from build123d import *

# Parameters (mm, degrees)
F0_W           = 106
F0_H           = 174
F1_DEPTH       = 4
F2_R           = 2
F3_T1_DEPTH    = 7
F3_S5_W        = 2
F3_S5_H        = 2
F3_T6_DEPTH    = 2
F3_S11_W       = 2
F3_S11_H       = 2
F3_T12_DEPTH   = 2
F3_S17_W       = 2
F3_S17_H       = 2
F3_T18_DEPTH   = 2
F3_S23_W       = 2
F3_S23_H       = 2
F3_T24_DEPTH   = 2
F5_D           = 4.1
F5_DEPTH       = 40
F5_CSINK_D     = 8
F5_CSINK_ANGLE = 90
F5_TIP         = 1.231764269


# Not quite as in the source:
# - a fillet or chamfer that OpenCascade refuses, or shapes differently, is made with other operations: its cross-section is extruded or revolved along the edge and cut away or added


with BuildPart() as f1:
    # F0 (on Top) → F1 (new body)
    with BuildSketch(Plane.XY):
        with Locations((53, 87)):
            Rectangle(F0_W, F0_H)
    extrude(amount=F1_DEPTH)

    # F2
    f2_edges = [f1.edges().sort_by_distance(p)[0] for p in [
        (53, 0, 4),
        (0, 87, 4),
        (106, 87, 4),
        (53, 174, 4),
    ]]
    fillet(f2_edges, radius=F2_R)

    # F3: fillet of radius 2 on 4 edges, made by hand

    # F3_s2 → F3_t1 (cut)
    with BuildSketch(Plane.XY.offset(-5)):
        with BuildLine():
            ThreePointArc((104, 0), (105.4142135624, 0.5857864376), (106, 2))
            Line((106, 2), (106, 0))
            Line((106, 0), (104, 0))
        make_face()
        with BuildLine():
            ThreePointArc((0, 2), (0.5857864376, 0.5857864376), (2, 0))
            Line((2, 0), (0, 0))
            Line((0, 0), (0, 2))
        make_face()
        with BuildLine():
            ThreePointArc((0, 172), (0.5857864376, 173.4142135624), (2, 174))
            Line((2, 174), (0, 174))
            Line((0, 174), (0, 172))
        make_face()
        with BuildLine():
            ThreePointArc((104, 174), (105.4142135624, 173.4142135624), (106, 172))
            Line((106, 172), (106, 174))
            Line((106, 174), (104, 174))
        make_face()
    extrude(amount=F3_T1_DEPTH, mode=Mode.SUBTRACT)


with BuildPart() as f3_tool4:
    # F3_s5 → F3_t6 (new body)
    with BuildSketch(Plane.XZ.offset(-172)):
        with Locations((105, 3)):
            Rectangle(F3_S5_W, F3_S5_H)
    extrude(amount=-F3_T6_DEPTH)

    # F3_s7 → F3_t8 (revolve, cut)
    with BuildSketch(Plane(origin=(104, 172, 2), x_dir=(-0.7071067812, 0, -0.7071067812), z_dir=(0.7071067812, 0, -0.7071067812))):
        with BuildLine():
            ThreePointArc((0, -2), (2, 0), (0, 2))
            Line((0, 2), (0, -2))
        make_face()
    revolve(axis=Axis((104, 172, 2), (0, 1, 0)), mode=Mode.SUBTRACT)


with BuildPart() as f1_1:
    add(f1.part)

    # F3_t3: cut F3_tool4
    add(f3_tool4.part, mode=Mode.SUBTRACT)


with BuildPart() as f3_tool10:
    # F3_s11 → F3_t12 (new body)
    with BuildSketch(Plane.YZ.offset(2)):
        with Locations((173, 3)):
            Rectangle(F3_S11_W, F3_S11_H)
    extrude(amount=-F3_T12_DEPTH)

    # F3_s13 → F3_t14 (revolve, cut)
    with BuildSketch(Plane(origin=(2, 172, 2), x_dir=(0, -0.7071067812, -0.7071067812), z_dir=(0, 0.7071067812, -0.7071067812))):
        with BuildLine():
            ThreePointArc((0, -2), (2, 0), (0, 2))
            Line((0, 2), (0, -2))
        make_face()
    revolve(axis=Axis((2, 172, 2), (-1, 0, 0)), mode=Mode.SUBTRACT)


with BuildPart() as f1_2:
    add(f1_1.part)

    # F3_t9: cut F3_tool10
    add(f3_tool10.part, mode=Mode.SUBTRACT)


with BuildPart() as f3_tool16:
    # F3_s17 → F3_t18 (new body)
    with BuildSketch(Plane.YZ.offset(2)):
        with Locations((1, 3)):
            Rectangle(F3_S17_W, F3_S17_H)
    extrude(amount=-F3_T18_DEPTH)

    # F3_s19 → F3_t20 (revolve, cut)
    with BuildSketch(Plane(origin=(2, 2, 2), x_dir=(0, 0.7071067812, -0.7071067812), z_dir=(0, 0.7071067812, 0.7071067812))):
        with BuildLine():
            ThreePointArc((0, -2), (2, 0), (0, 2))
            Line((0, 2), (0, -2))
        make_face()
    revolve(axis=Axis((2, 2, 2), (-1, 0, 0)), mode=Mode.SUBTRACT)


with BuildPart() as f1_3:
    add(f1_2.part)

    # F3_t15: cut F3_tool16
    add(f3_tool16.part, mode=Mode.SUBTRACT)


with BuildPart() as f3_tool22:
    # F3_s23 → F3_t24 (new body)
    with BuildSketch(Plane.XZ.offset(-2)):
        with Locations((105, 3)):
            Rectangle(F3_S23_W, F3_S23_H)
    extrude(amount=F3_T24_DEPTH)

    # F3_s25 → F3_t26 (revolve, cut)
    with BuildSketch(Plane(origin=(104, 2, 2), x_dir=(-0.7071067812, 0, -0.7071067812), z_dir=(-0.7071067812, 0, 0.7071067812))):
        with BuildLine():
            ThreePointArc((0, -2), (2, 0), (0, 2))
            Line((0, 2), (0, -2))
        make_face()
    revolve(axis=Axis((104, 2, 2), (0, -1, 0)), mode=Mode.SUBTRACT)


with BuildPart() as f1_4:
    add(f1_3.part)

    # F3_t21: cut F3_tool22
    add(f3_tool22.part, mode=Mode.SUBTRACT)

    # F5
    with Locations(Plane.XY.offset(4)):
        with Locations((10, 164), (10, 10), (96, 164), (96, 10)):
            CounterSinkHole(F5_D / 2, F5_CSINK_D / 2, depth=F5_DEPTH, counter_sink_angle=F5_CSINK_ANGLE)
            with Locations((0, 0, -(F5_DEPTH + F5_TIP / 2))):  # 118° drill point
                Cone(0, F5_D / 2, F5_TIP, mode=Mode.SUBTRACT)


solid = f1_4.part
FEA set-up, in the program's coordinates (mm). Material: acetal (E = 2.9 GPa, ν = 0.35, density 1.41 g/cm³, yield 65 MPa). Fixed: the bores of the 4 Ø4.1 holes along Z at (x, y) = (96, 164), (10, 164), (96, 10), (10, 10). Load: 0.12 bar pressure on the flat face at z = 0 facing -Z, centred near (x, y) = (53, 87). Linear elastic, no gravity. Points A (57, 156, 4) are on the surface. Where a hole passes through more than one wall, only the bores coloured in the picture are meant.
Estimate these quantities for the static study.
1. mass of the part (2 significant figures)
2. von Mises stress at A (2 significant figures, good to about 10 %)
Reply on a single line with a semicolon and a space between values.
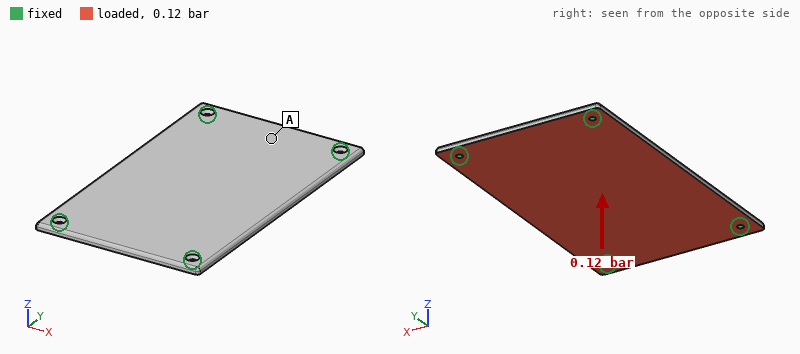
100 g; 2.8 MPa
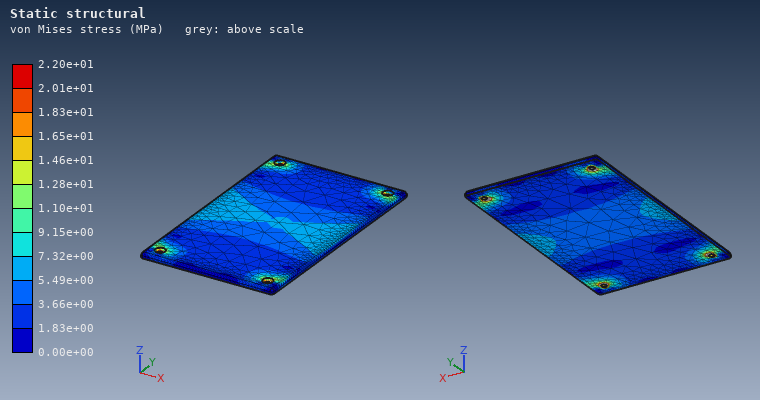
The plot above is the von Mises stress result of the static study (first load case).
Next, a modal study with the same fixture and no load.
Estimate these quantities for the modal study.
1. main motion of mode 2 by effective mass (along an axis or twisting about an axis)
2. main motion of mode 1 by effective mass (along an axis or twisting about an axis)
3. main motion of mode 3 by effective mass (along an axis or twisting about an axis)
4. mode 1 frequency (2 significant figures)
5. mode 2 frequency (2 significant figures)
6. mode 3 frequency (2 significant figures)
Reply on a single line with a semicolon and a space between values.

twisting about Y; along Z; twisting about X; 190 Hz; 320 Hz; 510 Hz
